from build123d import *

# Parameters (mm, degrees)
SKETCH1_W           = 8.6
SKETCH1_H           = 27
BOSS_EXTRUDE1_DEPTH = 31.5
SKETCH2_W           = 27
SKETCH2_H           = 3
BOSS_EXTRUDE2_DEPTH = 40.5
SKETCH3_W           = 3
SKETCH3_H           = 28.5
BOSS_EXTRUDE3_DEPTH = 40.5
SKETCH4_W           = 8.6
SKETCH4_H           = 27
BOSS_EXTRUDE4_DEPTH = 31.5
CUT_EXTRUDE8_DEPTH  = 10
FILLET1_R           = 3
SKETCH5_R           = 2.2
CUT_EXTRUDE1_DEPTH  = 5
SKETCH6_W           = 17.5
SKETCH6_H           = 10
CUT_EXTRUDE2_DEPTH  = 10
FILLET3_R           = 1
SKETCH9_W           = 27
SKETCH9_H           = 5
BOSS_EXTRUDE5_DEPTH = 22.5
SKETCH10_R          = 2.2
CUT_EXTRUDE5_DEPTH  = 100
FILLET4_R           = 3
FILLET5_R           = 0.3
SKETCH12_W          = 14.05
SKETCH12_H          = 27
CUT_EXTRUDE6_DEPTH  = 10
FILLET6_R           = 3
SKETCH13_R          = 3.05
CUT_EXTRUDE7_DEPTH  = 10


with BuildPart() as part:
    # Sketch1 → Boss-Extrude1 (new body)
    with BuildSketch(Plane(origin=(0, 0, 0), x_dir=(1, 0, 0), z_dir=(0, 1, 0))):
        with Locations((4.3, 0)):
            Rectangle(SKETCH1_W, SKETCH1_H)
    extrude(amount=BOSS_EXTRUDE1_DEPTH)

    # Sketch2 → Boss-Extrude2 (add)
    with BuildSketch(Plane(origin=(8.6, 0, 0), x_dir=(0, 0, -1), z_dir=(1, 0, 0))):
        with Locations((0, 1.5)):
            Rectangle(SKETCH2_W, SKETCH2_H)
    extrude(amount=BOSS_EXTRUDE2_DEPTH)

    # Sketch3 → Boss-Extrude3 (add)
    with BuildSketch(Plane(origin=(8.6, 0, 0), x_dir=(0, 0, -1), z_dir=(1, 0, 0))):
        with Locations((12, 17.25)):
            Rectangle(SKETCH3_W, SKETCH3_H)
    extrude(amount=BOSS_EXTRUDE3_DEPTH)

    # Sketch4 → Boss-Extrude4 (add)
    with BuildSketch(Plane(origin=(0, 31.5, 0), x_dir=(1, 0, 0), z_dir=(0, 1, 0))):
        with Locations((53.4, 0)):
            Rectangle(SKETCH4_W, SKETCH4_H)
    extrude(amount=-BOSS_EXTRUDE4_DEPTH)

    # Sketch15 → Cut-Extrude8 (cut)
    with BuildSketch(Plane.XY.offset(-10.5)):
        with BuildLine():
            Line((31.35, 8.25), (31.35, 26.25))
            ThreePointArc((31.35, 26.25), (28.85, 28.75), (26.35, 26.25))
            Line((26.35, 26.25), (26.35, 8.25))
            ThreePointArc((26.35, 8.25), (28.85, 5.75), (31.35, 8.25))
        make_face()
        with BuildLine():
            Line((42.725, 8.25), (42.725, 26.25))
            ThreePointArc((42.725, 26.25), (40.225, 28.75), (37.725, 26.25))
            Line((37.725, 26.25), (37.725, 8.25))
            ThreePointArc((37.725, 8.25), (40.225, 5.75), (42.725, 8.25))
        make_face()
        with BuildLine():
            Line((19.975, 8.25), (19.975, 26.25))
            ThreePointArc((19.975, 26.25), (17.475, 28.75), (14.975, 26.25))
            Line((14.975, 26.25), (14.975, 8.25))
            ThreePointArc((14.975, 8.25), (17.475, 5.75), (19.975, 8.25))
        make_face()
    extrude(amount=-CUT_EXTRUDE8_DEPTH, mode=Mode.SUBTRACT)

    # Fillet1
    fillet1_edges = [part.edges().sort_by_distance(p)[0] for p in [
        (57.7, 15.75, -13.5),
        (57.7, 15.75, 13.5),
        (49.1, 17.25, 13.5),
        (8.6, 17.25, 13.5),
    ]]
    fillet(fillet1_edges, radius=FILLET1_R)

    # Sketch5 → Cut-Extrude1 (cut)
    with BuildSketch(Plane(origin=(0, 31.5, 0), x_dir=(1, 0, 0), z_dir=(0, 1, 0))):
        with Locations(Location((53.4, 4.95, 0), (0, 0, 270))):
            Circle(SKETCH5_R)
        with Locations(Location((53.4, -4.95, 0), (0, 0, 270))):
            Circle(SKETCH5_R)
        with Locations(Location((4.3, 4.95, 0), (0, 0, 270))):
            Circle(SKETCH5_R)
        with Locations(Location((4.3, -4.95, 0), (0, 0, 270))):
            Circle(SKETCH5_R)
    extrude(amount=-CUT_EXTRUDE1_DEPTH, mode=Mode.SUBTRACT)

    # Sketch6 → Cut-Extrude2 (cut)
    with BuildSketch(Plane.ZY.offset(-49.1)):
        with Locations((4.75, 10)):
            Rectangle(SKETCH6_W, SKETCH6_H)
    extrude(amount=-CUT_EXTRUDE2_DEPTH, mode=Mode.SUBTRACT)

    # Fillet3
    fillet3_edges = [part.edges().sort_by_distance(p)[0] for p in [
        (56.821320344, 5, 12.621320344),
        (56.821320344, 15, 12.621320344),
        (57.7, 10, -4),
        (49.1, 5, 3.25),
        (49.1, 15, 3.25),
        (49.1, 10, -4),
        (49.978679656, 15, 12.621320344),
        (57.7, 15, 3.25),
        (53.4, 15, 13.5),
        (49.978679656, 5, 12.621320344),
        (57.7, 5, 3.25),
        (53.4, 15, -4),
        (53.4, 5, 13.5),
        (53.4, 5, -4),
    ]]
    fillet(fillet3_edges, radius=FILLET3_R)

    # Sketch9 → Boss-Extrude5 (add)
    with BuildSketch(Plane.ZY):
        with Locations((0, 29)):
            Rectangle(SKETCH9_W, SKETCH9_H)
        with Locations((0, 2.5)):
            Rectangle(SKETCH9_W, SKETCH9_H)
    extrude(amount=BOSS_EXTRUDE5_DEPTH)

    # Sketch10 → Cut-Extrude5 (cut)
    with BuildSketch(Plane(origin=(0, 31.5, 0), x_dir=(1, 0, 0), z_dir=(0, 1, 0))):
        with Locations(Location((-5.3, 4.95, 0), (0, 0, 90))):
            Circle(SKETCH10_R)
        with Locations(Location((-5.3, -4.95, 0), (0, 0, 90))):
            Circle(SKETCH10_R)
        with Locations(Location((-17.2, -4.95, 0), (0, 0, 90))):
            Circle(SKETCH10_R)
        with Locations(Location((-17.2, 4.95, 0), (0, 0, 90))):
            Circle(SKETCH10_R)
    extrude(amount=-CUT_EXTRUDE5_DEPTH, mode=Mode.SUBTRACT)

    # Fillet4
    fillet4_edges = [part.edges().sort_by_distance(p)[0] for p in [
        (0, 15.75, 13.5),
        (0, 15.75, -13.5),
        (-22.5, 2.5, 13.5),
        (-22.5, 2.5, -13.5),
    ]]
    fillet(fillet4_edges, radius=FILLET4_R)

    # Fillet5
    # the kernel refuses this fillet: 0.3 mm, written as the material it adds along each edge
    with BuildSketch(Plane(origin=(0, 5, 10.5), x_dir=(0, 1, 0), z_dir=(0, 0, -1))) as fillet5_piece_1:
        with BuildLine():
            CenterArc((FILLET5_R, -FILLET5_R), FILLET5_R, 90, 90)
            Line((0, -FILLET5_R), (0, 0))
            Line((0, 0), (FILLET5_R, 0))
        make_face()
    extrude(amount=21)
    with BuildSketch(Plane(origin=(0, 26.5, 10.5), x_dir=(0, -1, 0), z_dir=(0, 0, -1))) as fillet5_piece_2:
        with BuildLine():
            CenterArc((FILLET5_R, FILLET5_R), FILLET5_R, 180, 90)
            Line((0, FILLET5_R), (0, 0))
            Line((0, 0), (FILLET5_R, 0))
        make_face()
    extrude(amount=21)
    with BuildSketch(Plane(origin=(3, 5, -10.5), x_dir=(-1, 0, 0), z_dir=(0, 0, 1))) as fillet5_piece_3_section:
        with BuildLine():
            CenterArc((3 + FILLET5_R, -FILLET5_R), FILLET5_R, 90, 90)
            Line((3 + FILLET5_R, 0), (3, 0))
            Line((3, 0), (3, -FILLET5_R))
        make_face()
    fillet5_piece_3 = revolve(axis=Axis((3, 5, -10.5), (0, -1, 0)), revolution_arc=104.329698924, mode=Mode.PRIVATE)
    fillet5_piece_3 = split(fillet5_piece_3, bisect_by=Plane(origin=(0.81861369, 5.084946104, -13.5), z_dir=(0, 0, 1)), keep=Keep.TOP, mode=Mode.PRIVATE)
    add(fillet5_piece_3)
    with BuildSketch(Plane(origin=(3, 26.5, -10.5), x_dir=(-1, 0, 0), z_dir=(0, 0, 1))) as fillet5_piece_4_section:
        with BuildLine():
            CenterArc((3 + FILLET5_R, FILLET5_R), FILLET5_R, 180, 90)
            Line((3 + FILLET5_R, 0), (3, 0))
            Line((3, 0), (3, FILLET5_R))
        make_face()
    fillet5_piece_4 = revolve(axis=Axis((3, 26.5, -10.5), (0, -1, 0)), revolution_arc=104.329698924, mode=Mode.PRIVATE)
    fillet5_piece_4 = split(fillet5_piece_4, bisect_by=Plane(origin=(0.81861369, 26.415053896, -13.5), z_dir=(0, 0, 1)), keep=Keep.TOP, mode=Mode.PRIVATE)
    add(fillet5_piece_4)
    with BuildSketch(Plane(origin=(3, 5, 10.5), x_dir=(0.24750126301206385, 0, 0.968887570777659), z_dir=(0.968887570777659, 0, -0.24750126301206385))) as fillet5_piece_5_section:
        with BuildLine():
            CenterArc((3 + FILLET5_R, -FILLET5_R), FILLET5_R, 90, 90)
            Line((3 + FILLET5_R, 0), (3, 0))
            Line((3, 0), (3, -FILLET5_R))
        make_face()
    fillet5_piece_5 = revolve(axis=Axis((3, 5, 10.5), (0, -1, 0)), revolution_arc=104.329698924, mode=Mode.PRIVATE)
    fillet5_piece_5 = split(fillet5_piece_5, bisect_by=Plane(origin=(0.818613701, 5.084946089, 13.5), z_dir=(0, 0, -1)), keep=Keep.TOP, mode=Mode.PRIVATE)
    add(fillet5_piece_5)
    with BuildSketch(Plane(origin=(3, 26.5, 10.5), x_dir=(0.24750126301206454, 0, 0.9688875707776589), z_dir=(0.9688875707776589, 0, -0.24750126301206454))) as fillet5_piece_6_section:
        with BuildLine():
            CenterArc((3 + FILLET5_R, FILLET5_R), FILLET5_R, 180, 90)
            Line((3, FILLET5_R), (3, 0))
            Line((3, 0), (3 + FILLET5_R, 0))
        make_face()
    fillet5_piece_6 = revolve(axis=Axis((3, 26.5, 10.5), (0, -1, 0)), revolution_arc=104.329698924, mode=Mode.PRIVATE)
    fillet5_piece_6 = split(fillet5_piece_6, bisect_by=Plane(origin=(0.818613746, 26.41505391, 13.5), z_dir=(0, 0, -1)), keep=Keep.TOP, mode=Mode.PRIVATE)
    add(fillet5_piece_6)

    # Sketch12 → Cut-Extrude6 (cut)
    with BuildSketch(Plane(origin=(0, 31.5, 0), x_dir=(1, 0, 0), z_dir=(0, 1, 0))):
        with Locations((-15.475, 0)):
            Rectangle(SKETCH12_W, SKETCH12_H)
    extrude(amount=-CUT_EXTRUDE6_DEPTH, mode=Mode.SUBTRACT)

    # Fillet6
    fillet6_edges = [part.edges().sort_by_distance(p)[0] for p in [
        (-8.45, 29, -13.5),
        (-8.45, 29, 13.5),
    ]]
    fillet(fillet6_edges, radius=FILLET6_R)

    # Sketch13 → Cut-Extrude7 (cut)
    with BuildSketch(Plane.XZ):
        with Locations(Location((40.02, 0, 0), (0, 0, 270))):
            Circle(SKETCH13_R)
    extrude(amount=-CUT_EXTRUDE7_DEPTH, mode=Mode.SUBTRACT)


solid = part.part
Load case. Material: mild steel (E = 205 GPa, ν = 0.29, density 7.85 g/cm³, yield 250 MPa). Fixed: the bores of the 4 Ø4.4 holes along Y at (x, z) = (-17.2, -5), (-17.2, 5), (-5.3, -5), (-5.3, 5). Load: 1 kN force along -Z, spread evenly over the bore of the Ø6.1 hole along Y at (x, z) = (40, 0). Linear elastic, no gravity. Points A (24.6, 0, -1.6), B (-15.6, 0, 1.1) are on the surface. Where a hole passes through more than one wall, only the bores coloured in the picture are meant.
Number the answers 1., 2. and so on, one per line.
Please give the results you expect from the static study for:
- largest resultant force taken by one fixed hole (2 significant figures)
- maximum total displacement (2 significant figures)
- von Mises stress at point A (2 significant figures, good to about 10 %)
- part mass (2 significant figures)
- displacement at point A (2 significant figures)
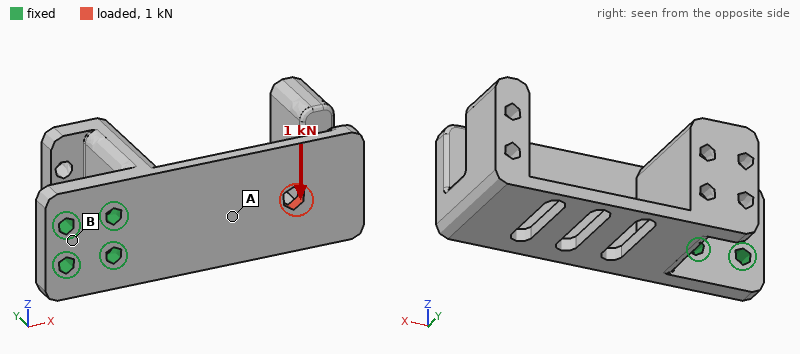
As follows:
1. 2.5 kN
2. 50 µm
3. 32 MPa
4. 170 g
5. 18 µm
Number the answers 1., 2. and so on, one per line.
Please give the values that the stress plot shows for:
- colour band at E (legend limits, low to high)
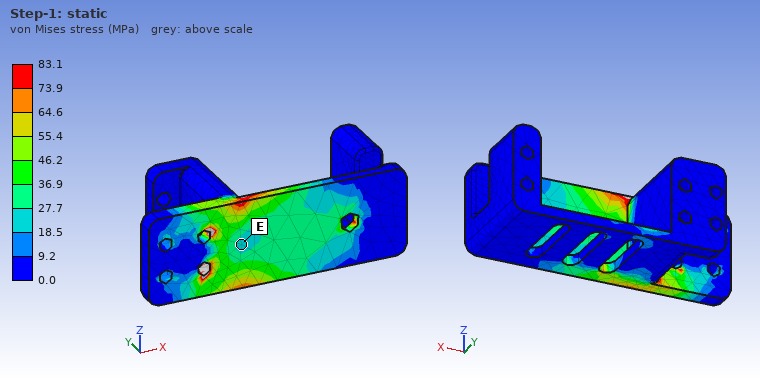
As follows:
1. 18.5 to 27.7 MPa
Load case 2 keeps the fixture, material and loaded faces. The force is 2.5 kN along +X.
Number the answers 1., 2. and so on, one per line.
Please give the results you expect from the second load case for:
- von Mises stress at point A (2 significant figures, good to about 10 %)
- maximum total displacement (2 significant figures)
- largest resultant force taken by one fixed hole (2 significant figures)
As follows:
1. 33 MPa
2. 29 µm
3. 1.1 kN
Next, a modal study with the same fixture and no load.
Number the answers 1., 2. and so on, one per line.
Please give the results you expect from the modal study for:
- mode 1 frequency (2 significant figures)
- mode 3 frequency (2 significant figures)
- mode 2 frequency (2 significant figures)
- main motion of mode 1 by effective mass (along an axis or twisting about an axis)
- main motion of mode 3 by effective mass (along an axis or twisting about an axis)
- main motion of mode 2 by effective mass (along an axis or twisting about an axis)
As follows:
1. 820 Hz
2. 3700 Hz
3. 1200 Hz
4. along Y
5. along Z
6. along Z
